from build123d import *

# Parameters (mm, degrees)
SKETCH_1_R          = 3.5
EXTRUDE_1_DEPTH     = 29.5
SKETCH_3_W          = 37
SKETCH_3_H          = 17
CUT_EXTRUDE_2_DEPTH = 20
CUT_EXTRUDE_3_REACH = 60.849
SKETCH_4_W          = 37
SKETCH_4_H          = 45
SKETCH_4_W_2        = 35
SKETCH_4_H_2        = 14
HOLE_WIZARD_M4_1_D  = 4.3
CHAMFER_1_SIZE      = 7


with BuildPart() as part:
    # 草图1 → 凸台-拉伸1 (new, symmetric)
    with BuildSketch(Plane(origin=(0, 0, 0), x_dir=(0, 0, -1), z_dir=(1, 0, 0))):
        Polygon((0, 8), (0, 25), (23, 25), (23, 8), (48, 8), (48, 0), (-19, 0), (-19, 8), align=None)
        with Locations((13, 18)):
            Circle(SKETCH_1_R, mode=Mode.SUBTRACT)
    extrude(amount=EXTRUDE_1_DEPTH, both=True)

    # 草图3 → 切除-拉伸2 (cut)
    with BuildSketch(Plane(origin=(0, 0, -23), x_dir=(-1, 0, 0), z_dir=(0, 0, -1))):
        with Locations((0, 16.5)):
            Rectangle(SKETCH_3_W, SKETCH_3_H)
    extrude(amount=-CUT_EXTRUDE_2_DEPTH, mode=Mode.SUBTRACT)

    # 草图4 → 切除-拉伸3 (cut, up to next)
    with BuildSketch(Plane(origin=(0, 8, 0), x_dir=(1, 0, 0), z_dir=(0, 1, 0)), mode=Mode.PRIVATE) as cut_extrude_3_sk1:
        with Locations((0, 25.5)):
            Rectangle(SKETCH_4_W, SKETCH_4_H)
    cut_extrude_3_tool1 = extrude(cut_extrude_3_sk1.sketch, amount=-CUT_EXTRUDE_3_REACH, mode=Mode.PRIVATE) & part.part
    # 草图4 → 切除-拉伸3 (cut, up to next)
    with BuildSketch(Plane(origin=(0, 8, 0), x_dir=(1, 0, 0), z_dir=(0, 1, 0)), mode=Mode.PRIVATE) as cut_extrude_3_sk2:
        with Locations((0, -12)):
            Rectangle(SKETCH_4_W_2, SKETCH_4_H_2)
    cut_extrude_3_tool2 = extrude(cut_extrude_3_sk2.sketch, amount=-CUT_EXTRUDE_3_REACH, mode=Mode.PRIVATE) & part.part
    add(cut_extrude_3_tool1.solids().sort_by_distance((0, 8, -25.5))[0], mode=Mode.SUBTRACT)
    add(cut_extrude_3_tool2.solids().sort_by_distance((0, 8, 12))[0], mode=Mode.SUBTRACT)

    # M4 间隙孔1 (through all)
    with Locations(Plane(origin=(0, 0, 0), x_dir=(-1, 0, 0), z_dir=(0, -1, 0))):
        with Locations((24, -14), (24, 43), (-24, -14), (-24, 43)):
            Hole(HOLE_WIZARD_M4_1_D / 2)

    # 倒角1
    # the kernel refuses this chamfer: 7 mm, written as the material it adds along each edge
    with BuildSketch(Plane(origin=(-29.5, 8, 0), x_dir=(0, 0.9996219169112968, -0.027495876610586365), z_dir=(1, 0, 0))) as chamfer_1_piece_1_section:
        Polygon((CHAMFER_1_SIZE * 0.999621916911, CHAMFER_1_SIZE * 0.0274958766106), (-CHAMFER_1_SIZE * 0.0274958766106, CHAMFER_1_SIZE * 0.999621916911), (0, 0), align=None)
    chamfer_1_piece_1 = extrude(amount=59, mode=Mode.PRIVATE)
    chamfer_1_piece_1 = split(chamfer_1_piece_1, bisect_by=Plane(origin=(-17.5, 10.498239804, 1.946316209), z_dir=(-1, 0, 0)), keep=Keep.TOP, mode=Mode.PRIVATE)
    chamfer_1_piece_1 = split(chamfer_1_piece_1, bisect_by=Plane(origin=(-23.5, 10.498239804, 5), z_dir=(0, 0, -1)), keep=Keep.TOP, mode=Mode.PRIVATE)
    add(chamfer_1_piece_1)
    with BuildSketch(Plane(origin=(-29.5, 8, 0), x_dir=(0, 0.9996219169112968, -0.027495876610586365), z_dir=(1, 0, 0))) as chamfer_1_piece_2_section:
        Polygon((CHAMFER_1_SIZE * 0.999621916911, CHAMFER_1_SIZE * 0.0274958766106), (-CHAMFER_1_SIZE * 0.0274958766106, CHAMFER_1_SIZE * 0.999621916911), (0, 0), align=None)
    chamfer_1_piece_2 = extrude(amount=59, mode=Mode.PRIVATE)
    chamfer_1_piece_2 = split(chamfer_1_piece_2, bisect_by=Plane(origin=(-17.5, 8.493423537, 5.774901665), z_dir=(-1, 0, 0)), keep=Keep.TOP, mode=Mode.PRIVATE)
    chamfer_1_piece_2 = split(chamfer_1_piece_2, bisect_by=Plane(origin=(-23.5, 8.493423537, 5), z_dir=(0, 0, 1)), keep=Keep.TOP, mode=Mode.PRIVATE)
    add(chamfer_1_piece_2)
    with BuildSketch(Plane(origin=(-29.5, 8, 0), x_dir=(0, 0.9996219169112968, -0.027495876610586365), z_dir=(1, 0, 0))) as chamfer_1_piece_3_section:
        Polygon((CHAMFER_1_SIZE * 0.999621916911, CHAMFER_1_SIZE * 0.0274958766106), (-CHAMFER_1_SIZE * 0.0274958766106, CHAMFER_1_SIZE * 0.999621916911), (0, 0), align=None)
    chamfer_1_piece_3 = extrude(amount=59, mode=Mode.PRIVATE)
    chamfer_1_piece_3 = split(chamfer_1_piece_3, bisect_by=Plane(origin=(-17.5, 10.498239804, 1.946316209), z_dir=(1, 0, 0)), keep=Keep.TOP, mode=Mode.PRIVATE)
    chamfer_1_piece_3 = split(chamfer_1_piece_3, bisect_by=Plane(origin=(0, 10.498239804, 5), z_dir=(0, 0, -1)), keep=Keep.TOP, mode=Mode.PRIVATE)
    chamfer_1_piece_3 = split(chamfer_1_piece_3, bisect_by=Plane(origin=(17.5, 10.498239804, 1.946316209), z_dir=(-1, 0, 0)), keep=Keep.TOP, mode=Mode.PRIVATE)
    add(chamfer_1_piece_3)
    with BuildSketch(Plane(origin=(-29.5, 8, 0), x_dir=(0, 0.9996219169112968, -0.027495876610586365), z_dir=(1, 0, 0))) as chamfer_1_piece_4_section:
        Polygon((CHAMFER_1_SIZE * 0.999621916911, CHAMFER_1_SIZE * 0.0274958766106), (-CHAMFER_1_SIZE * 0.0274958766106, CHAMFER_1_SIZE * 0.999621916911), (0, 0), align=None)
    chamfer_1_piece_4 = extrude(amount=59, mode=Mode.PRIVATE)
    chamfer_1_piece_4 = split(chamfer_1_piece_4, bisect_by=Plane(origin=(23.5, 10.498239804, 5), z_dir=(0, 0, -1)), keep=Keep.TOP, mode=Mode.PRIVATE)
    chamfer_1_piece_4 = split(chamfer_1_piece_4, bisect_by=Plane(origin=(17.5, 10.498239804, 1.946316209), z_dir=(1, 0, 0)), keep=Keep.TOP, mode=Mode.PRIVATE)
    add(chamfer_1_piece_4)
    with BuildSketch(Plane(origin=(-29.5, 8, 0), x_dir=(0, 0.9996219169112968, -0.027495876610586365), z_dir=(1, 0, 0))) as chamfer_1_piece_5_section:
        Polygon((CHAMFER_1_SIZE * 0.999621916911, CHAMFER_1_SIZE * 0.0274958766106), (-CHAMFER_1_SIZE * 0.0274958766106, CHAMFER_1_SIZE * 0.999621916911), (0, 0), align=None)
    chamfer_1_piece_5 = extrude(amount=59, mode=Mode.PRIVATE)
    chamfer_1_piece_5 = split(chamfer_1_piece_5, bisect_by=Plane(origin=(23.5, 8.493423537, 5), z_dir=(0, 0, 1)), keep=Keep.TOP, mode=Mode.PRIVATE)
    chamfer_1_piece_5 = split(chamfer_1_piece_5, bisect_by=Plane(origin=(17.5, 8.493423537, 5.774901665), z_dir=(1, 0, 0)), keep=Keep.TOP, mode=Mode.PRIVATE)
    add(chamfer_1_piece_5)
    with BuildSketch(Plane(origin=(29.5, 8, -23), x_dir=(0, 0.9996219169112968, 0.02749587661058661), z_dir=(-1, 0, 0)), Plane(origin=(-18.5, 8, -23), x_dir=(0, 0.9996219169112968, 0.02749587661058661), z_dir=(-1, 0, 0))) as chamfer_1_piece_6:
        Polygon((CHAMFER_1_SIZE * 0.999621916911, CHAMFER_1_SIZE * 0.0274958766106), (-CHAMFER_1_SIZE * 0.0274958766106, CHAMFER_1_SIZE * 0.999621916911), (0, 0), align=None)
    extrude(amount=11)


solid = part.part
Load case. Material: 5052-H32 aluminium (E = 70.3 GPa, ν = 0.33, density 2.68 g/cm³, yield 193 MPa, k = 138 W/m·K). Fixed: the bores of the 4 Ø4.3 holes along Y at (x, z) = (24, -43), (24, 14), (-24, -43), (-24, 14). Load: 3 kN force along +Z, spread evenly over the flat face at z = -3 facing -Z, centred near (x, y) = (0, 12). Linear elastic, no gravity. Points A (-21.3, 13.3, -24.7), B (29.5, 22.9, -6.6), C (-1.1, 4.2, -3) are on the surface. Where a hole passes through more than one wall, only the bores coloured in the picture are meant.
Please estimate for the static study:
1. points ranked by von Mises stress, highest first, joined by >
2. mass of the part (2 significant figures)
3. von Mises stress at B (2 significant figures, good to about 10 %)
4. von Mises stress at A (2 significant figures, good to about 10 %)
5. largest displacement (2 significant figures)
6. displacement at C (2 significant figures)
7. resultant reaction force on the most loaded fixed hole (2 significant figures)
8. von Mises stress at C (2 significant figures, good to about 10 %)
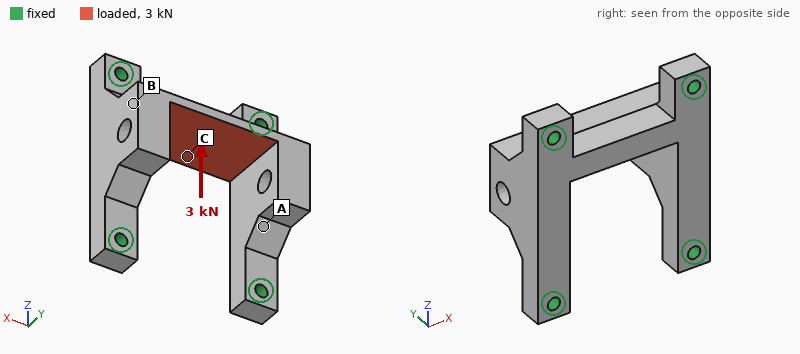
C > A > B
68 g
7.3 MPa
14 MPa
85 µm
23 µm
1.2 kN
44 MPa
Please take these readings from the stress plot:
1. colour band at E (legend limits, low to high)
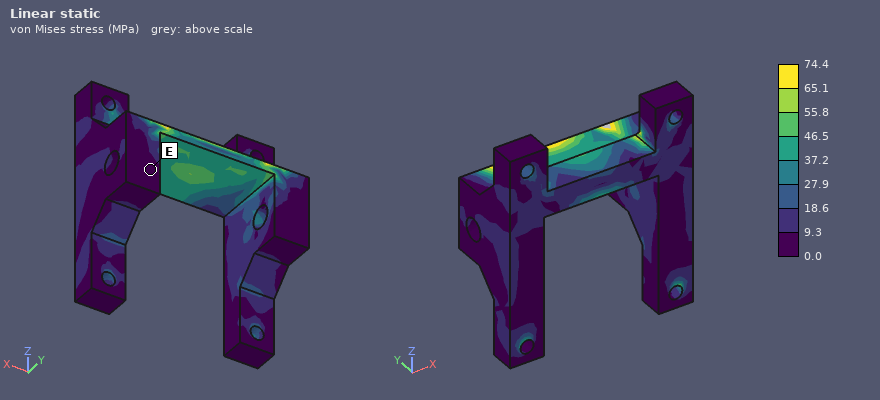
0.0 to 9.3 MPa
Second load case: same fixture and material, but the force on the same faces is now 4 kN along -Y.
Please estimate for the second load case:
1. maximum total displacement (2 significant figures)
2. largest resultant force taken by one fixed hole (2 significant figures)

61 µm
1.6 kN
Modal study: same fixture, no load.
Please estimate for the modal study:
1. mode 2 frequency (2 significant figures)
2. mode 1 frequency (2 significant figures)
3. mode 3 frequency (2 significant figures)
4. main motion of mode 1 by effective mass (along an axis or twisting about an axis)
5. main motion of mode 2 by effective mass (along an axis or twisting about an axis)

10 kHz
9000 Hz
12 kHz
along X
along Y
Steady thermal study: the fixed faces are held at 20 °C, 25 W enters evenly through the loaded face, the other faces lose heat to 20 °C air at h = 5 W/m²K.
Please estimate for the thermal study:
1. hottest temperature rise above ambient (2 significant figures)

17 K
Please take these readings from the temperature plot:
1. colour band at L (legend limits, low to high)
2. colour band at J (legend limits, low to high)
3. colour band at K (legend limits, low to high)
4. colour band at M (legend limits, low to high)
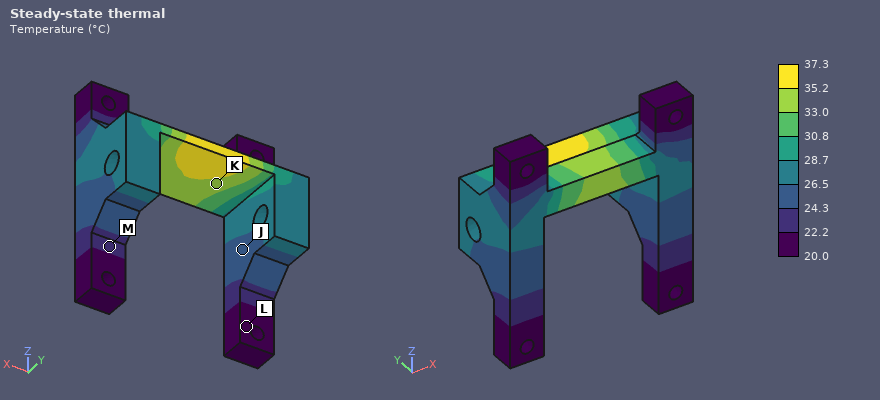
20.0 to 22.2 °C
24.3 to 26.5 °C
33.0 to 35.2 °C
22.2 to 24.3 °C
